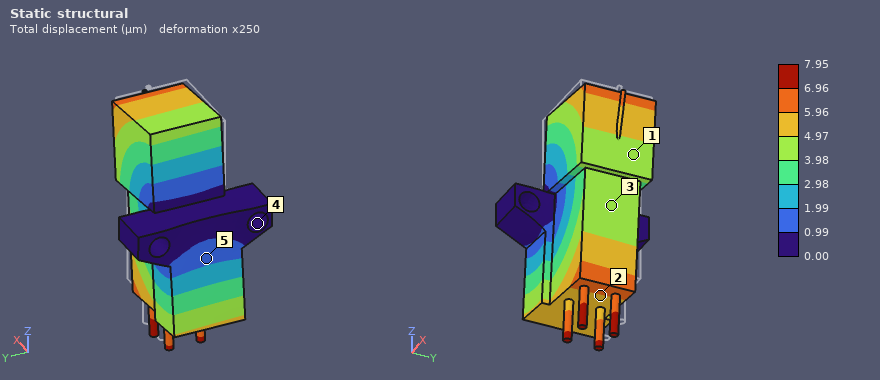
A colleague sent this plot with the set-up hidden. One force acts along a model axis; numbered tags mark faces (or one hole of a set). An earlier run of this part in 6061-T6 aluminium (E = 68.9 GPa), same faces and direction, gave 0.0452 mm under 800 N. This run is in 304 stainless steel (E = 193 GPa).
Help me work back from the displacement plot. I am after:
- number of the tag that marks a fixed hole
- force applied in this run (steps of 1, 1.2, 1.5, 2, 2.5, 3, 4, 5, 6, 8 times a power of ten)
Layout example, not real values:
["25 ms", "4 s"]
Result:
["4", "400 N"]
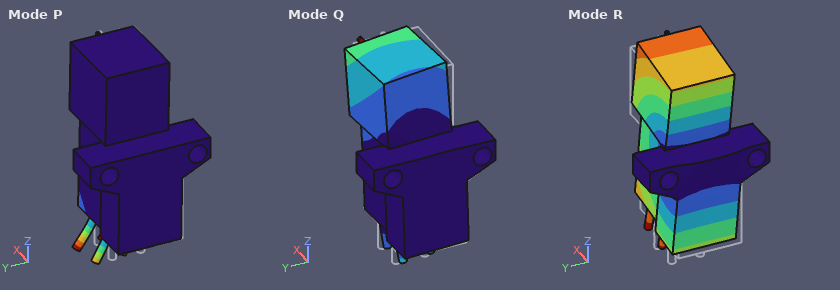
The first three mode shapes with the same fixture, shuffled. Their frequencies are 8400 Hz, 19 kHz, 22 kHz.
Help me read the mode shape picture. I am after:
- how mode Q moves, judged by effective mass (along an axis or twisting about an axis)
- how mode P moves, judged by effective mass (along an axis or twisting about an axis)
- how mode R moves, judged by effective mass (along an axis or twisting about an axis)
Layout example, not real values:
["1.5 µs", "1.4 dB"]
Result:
["along Y", "along Y", "along Z"]
